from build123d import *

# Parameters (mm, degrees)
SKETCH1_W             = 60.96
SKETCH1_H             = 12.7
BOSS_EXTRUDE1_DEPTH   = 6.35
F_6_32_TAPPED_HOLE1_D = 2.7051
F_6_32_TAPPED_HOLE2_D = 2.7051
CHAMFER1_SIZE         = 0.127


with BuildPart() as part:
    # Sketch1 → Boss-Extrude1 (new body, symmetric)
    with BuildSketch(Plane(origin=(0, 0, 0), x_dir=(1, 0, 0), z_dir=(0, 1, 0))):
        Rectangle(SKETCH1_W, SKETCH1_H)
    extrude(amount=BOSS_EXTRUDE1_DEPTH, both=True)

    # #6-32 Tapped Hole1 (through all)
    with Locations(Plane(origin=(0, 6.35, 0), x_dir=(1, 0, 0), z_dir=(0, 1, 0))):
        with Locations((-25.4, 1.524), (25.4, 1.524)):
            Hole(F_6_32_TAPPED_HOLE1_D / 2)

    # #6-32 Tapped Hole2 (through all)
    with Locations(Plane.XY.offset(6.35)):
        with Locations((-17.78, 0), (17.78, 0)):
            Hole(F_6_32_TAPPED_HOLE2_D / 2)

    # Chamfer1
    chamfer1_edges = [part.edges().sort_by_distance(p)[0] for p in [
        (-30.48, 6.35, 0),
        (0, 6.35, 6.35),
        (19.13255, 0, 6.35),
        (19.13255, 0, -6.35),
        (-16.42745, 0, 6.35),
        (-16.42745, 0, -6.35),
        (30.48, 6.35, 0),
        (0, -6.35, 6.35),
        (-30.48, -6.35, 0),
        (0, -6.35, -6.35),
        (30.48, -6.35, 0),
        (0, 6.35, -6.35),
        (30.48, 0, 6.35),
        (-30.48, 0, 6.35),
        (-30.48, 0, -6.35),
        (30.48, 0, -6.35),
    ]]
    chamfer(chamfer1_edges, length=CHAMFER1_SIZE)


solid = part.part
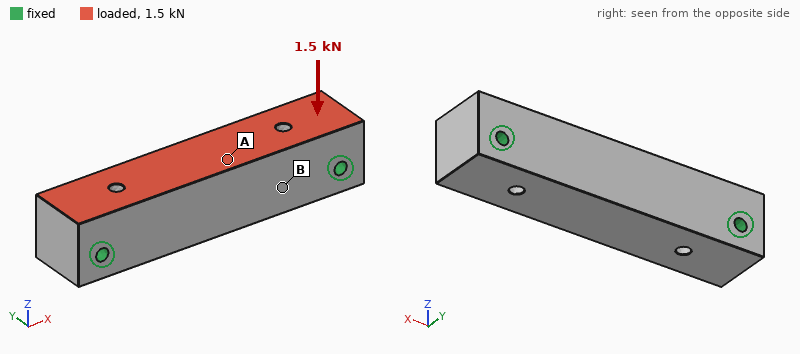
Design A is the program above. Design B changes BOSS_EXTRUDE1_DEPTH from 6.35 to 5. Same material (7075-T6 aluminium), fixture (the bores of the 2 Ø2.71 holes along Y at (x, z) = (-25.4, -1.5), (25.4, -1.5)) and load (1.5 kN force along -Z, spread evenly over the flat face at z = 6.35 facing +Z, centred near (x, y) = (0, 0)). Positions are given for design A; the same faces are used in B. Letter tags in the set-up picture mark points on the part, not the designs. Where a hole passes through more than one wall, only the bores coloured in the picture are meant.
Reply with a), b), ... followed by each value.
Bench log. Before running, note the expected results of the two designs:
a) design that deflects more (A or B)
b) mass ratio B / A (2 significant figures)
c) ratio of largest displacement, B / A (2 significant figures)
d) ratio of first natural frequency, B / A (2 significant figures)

a) B
b) 0.78
c) 1.3
d) 1.00
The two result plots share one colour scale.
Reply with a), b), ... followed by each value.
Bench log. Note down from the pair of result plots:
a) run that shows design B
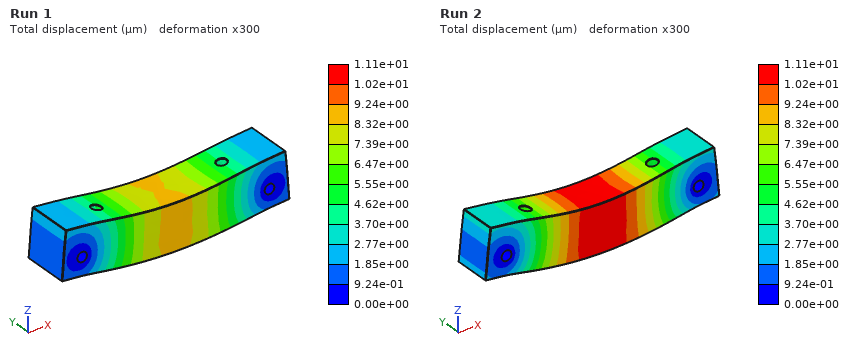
a) Run 2
